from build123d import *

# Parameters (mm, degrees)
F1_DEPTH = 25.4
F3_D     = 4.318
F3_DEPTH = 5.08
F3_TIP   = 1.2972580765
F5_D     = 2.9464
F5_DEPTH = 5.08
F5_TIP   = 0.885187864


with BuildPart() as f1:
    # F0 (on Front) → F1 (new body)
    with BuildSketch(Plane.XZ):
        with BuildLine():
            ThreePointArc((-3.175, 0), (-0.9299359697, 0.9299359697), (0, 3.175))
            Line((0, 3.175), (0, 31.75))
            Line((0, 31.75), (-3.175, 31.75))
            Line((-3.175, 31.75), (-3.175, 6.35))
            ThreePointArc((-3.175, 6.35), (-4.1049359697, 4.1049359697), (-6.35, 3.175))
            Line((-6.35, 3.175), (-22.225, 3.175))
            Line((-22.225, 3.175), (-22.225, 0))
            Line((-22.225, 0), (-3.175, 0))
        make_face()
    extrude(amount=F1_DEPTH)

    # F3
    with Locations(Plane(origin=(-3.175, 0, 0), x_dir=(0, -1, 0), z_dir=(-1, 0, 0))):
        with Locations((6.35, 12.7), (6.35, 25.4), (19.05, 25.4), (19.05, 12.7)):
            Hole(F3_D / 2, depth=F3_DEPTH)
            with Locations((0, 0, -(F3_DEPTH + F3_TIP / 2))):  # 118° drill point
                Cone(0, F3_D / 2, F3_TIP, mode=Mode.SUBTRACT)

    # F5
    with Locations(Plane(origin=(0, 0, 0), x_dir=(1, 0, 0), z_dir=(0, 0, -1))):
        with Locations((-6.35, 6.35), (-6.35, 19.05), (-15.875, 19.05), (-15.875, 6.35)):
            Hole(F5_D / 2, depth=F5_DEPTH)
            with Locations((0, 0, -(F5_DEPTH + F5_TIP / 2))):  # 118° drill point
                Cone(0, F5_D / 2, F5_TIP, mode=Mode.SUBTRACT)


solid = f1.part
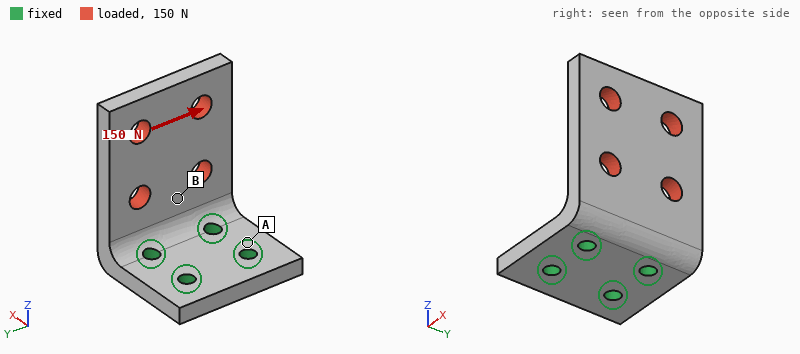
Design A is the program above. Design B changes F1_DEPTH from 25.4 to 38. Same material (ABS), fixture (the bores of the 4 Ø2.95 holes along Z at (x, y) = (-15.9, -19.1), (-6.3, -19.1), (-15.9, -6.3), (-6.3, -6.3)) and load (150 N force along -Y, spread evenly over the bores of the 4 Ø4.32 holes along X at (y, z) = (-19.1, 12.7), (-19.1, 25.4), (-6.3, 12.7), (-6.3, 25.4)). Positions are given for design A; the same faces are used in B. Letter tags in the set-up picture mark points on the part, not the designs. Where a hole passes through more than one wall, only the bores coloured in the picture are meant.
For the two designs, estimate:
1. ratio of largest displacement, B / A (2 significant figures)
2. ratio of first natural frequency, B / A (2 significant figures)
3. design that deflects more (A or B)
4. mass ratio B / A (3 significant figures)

1.1
0.94
B
1.53
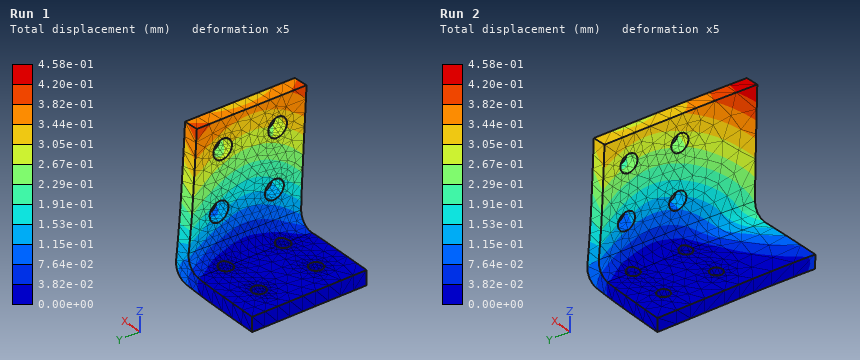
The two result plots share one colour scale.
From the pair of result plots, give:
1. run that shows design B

Run 2
